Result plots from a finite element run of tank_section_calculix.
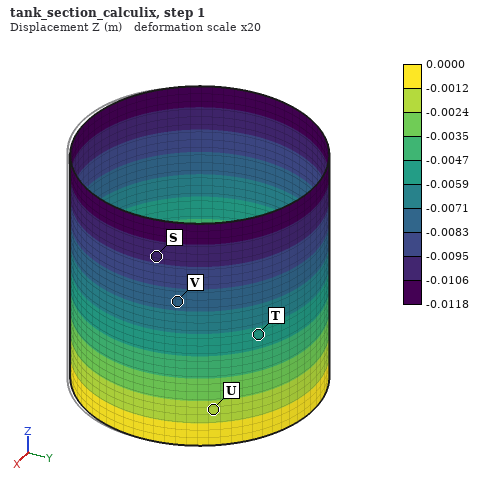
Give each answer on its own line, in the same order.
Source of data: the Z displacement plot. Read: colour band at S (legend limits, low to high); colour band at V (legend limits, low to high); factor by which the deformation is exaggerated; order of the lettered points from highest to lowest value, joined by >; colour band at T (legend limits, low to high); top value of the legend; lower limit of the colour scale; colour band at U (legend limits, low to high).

-0.0106 to -0.0095 m
-0.0083 to -0.0071 m
20
U > T > V > S
-0.0059 to -0.0047 m
0.0000 m
-0.0118 m
-0.0024 to -0.0012 m
